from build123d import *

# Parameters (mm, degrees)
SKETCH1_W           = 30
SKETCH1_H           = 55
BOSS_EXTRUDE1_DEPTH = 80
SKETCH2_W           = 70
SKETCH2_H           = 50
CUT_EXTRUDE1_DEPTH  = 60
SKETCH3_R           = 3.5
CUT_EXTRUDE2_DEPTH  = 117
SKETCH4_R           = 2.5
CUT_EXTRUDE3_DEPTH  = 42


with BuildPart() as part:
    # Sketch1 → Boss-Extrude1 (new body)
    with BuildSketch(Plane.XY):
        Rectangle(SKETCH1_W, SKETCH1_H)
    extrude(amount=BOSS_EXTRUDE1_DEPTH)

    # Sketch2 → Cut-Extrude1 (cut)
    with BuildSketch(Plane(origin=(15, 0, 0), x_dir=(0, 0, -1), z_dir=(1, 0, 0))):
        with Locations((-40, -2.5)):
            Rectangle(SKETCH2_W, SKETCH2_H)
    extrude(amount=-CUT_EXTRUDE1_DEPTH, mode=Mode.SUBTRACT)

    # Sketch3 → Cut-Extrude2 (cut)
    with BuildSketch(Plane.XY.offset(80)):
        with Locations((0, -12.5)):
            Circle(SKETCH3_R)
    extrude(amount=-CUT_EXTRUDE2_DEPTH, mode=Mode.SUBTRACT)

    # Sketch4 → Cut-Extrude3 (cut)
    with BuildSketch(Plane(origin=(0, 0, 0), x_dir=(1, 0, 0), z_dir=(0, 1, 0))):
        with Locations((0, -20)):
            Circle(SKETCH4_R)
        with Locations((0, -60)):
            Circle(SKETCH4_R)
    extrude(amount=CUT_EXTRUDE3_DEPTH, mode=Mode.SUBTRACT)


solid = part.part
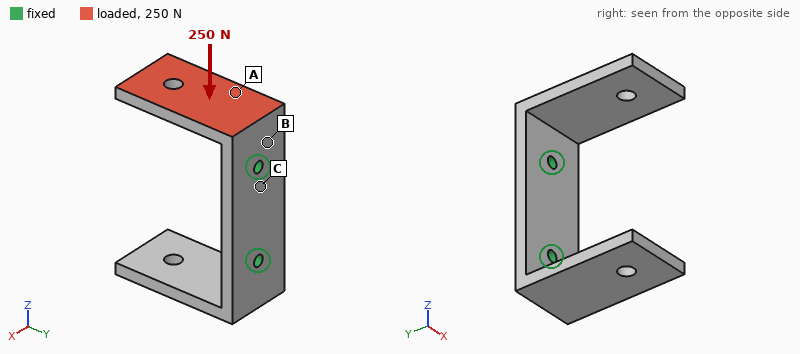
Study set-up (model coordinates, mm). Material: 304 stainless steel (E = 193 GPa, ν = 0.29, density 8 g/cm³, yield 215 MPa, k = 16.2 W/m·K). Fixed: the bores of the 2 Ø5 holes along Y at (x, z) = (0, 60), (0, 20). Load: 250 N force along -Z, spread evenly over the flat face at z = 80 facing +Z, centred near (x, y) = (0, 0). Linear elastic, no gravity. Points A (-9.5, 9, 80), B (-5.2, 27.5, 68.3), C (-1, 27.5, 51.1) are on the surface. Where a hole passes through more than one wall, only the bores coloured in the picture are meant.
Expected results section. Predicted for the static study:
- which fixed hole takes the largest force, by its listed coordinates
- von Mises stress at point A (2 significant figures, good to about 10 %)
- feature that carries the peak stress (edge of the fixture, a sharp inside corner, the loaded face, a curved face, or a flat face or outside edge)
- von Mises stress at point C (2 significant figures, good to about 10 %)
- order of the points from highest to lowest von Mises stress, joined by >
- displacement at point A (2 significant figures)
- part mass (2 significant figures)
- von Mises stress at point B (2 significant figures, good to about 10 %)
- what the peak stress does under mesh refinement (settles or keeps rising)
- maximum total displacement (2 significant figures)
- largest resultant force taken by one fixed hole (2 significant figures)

(0, 60)
23 MPa
edge of the fixture
9.0 MPa
B > A > C
0.043 mm
210 g
44 MPa
keeps rising
0.16 mm
220 N
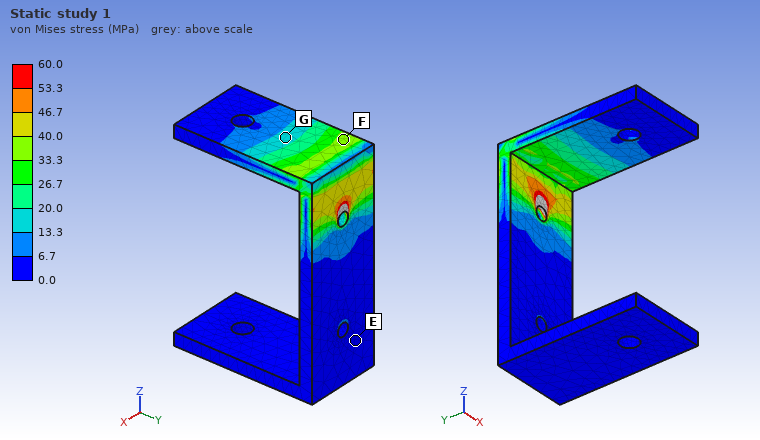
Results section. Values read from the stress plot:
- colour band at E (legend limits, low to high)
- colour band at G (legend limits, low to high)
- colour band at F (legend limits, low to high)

0.0 to 6.7 MPa
13.3 to 20.0 MPa
33.3 to 40.0 MPa
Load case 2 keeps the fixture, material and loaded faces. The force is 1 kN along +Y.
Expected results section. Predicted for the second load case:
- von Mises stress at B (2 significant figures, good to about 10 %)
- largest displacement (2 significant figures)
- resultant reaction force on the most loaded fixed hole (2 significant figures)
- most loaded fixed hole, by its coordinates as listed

88 MPa
0.22 mm
1.1 kN
(0, 60)
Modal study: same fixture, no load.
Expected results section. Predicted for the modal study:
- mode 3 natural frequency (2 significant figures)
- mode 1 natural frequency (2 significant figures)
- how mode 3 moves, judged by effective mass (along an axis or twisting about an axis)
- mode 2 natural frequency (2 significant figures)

1500 Hz
960 Hz
along X
970 Hz
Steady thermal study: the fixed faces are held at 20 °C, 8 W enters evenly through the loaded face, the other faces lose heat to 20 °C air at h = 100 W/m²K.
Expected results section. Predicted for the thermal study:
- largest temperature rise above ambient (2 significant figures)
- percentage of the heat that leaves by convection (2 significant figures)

28 K
82 %
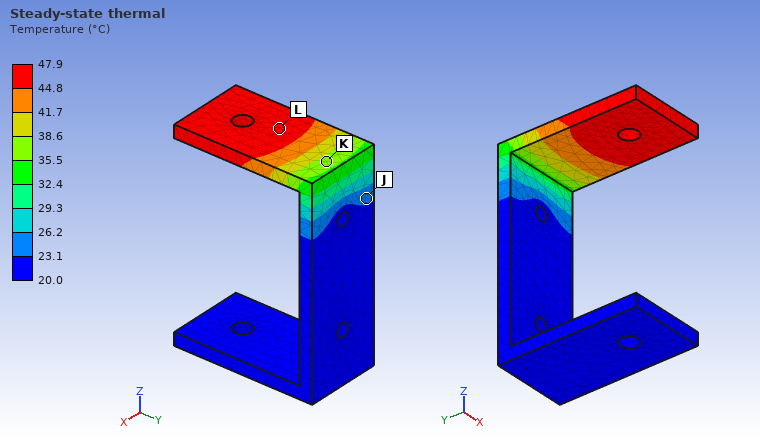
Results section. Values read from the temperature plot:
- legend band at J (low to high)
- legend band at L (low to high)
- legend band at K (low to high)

23.1 to 26.2 °C
44.8 to 47.9 °C
35.5 to 38.6 °C
